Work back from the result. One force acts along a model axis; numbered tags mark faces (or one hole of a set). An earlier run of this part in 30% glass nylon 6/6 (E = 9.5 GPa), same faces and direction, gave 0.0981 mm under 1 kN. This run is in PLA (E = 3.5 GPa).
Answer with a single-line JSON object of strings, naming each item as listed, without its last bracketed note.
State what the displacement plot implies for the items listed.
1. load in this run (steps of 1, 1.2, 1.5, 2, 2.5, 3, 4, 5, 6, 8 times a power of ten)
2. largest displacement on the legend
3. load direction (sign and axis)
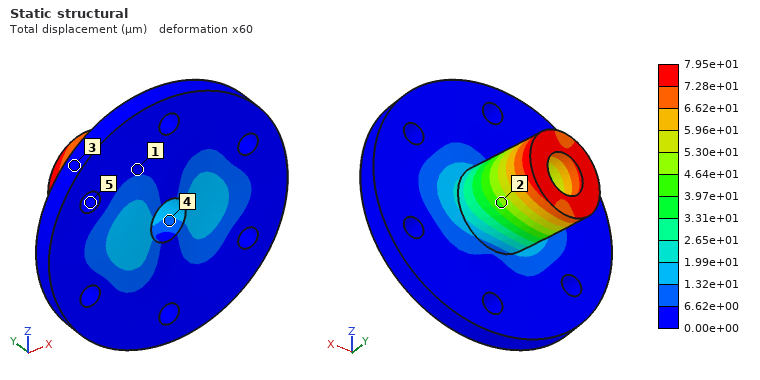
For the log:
{"load in this run": "300 N", "largest displacement on the legend": "7.95e+01 µm", "load direction": "-X"}
